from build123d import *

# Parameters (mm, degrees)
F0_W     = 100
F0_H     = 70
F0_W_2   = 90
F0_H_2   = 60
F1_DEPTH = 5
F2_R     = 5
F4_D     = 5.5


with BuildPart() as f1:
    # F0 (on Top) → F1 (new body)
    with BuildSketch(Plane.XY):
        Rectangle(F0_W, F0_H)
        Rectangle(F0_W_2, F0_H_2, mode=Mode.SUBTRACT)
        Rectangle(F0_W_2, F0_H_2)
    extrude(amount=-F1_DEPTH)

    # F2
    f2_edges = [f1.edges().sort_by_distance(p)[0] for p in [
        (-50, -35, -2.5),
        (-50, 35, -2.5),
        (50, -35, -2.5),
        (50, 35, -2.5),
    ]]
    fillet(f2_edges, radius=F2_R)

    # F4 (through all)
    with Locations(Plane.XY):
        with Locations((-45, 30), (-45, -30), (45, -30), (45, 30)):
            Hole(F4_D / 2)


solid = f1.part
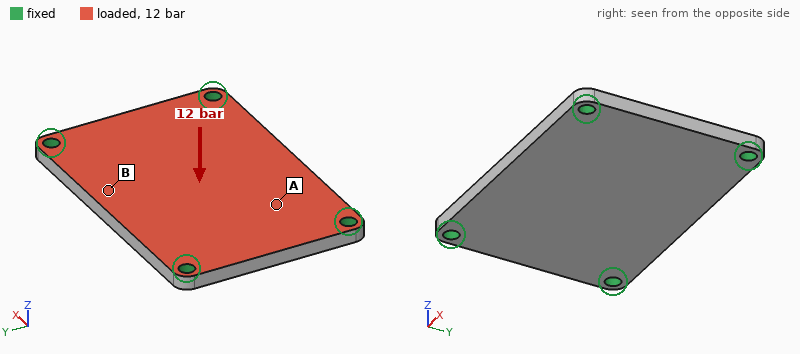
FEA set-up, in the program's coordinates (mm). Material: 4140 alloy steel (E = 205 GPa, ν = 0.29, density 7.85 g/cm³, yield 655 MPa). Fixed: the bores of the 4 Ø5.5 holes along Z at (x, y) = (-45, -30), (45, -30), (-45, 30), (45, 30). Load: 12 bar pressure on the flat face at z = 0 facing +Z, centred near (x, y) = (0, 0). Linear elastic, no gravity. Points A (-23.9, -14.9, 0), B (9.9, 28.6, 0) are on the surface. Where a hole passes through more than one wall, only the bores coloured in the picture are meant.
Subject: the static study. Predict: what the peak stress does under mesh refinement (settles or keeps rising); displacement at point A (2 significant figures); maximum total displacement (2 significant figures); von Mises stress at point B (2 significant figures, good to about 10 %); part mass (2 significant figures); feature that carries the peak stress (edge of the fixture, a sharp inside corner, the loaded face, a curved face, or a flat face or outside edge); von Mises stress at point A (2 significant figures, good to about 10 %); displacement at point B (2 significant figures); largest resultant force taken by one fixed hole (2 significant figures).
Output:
keeps rising
0.092 mm
0.15 mm
110 MPa
270 g
edge of the fixture
48 MPa
0.12 mm
2.1 kN
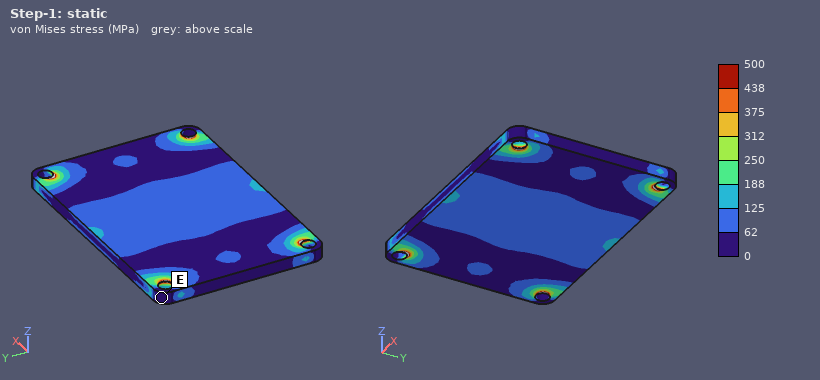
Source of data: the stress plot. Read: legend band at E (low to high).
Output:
0 to 62 MPa
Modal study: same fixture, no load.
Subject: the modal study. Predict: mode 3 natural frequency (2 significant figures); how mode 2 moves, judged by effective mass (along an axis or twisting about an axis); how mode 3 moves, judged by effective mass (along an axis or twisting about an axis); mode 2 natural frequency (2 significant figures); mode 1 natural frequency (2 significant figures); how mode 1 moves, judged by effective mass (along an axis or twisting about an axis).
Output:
6400 Hz
twisting about X
twisting about Y
4300 Hz
2700 Hz
along Z
